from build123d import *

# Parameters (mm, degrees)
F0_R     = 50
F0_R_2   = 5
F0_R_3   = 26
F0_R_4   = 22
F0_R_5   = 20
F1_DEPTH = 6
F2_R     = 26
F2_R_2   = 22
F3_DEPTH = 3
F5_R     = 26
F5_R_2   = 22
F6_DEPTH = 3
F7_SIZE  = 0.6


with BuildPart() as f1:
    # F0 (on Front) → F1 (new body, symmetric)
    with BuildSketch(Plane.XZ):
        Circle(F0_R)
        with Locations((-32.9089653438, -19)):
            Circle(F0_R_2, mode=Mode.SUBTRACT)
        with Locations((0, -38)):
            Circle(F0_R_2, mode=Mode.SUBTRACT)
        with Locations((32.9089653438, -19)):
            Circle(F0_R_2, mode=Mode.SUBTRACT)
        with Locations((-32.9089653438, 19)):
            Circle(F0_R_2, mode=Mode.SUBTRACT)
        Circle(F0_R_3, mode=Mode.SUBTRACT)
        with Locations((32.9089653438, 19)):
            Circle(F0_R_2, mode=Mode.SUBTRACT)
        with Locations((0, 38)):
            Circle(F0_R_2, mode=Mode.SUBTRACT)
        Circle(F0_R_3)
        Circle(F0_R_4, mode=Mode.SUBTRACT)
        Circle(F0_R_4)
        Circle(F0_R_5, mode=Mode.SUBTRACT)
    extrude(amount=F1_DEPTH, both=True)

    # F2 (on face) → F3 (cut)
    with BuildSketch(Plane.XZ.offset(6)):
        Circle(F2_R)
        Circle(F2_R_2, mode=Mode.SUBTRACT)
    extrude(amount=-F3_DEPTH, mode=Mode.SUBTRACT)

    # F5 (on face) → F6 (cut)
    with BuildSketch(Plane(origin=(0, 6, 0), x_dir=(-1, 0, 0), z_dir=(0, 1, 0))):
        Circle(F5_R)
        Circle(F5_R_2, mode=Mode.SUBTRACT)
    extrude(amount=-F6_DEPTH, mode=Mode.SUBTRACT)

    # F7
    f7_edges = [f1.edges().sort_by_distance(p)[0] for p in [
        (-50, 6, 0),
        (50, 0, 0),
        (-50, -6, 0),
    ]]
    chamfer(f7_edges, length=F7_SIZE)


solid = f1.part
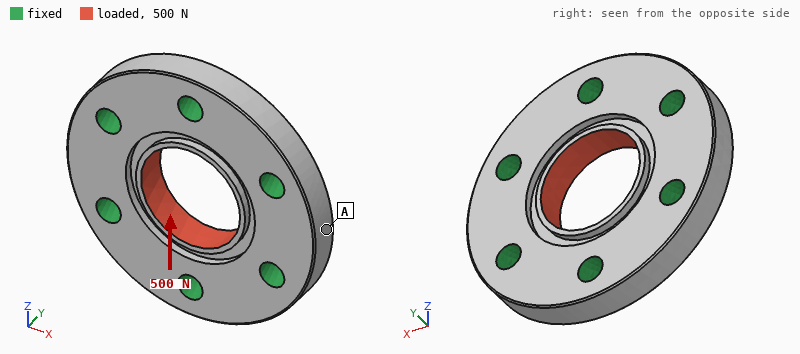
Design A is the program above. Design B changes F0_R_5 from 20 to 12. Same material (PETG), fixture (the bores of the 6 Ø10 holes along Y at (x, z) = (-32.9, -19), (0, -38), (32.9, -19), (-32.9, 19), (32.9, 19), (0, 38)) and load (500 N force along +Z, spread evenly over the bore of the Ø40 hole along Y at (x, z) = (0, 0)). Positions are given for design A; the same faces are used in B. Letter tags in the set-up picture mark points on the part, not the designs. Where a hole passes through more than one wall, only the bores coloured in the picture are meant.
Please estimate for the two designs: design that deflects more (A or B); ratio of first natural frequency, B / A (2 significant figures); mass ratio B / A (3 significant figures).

A
0.68
1.14
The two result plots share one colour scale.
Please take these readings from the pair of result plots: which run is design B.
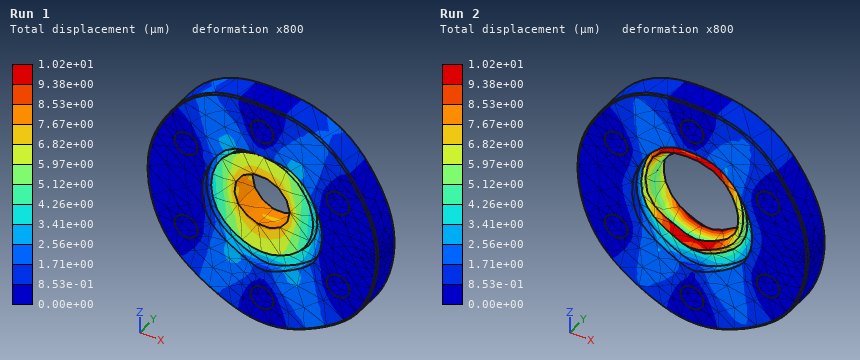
Run 1
